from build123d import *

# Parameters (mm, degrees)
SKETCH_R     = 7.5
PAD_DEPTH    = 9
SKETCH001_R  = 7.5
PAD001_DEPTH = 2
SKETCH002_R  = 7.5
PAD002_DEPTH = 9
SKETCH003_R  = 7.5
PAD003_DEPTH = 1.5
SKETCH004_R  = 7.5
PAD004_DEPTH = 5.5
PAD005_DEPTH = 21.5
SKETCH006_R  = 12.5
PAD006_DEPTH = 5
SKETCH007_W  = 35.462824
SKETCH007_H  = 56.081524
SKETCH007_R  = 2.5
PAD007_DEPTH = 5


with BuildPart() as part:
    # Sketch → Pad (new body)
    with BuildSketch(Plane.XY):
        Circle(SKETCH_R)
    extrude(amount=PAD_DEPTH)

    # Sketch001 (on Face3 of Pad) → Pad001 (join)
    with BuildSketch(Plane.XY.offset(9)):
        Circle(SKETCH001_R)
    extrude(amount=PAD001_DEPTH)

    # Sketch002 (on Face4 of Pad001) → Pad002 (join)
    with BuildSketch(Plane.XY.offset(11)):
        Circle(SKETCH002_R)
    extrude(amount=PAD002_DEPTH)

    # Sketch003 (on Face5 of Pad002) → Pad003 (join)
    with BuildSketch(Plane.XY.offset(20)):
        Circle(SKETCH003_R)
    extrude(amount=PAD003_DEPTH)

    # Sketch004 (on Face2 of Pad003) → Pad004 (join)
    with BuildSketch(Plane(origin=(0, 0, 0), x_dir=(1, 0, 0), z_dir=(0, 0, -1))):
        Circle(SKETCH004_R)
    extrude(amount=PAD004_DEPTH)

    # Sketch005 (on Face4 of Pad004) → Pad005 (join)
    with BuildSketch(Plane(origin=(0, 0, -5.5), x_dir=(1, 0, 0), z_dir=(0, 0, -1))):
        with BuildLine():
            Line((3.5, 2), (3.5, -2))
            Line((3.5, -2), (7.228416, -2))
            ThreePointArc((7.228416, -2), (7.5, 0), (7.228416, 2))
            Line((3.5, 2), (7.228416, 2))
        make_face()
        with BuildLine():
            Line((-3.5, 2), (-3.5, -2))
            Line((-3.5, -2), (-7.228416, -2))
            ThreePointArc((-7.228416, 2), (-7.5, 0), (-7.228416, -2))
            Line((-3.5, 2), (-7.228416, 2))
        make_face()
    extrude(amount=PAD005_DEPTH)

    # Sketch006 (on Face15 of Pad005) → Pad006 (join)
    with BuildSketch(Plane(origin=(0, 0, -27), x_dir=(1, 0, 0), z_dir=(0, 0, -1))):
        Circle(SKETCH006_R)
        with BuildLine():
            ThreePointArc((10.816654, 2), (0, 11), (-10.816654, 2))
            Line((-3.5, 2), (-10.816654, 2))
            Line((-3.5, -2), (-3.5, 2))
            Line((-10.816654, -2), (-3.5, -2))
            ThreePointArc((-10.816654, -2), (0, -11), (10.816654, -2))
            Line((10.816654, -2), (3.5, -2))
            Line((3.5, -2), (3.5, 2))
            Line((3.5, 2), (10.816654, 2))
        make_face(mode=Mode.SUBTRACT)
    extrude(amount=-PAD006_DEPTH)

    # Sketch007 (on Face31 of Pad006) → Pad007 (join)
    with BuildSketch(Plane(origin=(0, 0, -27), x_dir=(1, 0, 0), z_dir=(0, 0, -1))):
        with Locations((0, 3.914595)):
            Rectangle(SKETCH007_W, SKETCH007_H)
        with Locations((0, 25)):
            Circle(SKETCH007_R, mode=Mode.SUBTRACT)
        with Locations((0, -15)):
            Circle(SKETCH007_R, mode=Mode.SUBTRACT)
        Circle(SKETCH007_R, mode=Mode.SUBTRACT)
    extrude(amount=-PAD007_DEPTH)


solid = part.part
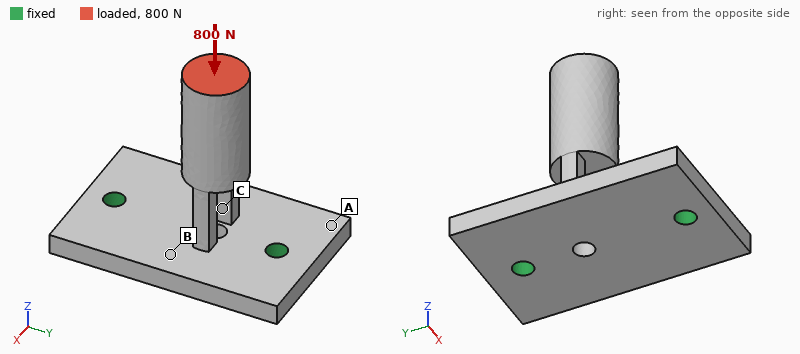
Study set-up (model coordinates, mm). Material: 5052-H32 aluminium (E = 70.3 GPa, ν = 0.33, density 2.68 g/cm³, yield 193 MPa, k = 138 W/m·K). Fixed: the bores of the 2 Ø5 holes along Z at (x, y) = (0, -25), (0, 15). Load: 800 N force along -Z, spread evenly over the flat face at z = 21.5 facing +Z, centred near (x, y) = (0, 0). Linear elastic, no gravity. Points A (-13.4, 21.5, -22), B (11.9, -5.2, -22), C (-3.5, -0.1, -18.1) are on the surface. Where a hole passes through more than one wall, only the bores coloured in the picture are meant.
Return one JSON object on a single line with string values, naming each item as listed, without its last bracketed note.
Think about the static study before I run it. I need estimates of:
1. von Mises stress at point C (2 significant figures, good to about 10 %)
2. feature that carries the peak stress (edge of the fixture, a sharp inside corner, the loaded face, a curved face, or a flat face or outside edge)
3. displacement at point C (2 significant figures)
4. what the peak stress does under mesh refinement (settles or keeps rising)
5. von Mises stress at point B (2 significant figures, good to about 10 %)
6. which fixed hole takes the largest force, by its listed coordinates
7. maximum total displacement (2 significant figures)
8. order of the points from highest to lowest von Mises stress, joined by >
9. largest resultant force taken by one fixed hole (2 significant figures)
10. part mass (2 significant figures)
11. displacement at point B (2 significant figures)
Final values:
{"von Mises stress at point C": "24 MPa", "feature that carries the peak stress": "edge of the fixture", "displacement at point C": "15 µm", "what the peak stress does under mesh refinement": "keeps rising", "von Mises stress at point B": "15 MPa", "which fixed hole takes the largest force, by its listed coordinates": "(0, 15)", "maximum total displacement": "32 µm", "order of the points from highest to lowest von Mises stress, joined by >": "C > B > A", "largest resultant force taken by one fixed hole": "540 N", "part mass": "40 g", "displacement at point B": "13 µm"}
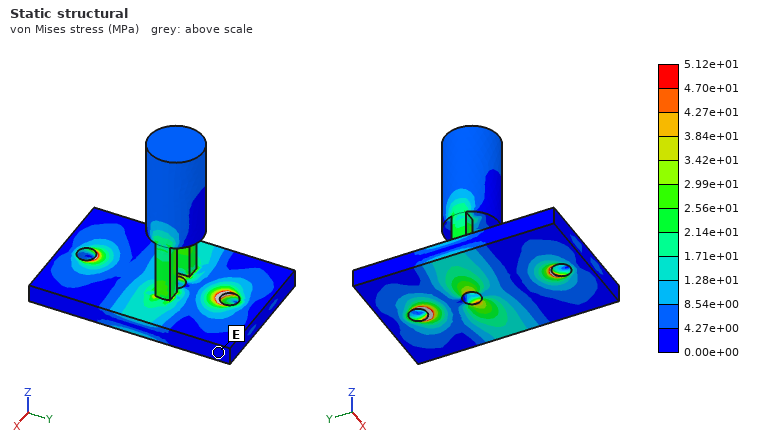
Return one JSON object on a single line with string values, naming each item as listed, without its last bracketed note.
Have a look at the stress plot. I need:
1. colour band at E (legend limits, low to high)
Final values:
{"colour band at E": "0.00e+00 to 4.27e+00 MPa"}
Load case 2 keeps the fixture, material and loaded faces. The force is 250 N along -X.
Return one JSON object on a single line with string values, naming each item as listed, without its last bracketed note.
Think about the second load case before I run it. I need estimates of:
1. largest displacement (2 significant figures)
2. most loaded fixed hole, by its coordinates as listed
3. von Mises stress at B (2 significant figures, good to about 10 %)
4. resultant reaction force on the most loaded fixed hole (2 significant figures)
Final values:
{"largest displacement": "0.27 mm", "most loaded fixed hole, by its coordinates as listed": "(0, 15)", "von Mises stress at B": "18 MPa", "resultant reaction force on the most loaded fixed hole": "160 N"}
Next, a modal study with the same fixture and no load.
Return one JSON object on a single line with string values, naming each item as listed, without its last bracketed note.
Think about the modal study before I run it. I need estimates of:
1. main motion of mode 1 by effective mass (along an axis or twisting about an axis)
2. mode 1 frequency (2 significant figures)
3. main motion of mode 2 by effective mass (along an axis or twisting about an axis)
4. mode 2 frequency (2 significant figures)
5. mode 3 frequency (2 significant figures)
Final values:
{"main motion of mode 1 by effective mass": "along Y", "mode 1 frequency": "720 Hz", "main motion of mode 2 by effective mass": "along X", "mode 2 frequency": "1800 Hz", "mode 3 frequency": "4100 Hz"}
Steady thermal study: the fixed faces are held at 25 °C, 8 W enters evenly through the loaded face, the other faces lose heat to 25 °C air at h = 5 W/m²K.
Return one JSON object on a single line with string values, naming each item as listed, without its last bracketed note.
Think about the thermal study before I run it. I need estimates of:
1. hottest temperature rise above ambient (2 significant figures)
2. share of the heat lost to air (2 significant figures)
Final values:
{"hottest temperature rise above ambient": "46 K", "share of the heat lost to air": "4.8 %"}
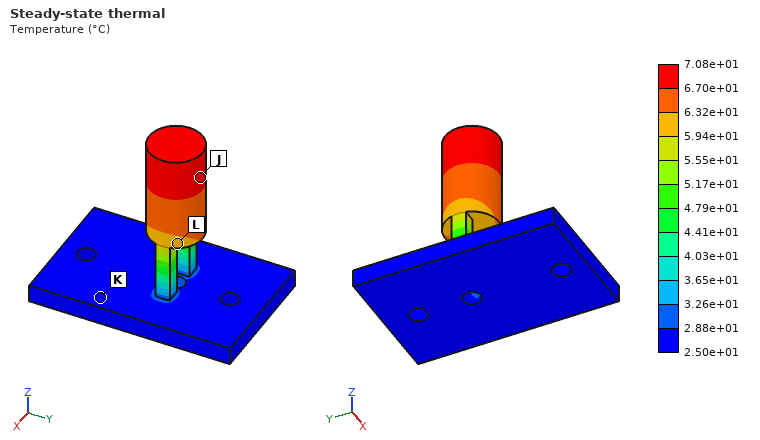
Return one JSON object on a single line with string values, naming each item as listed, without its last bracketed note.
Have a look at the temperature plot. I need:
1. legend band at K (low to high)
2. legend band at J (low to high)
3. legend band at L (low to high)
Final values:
{"legend band at K": "2.50e+01 to 2.88e+01 °C", "legend band at J": "6.70e+01 to 7.08e+01 °C", "legend band at L": "5.94e+01 to 6.32e+01 °C"}
